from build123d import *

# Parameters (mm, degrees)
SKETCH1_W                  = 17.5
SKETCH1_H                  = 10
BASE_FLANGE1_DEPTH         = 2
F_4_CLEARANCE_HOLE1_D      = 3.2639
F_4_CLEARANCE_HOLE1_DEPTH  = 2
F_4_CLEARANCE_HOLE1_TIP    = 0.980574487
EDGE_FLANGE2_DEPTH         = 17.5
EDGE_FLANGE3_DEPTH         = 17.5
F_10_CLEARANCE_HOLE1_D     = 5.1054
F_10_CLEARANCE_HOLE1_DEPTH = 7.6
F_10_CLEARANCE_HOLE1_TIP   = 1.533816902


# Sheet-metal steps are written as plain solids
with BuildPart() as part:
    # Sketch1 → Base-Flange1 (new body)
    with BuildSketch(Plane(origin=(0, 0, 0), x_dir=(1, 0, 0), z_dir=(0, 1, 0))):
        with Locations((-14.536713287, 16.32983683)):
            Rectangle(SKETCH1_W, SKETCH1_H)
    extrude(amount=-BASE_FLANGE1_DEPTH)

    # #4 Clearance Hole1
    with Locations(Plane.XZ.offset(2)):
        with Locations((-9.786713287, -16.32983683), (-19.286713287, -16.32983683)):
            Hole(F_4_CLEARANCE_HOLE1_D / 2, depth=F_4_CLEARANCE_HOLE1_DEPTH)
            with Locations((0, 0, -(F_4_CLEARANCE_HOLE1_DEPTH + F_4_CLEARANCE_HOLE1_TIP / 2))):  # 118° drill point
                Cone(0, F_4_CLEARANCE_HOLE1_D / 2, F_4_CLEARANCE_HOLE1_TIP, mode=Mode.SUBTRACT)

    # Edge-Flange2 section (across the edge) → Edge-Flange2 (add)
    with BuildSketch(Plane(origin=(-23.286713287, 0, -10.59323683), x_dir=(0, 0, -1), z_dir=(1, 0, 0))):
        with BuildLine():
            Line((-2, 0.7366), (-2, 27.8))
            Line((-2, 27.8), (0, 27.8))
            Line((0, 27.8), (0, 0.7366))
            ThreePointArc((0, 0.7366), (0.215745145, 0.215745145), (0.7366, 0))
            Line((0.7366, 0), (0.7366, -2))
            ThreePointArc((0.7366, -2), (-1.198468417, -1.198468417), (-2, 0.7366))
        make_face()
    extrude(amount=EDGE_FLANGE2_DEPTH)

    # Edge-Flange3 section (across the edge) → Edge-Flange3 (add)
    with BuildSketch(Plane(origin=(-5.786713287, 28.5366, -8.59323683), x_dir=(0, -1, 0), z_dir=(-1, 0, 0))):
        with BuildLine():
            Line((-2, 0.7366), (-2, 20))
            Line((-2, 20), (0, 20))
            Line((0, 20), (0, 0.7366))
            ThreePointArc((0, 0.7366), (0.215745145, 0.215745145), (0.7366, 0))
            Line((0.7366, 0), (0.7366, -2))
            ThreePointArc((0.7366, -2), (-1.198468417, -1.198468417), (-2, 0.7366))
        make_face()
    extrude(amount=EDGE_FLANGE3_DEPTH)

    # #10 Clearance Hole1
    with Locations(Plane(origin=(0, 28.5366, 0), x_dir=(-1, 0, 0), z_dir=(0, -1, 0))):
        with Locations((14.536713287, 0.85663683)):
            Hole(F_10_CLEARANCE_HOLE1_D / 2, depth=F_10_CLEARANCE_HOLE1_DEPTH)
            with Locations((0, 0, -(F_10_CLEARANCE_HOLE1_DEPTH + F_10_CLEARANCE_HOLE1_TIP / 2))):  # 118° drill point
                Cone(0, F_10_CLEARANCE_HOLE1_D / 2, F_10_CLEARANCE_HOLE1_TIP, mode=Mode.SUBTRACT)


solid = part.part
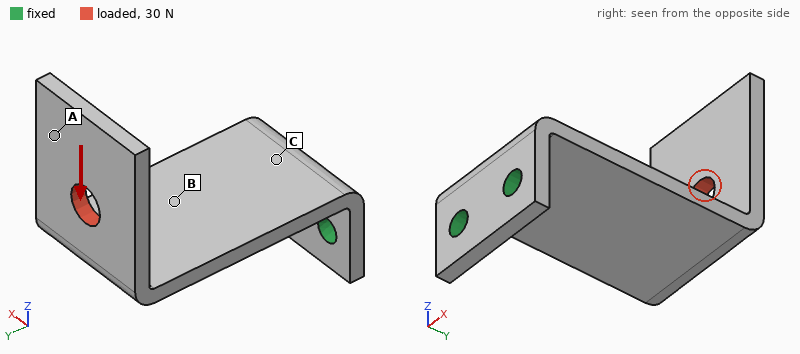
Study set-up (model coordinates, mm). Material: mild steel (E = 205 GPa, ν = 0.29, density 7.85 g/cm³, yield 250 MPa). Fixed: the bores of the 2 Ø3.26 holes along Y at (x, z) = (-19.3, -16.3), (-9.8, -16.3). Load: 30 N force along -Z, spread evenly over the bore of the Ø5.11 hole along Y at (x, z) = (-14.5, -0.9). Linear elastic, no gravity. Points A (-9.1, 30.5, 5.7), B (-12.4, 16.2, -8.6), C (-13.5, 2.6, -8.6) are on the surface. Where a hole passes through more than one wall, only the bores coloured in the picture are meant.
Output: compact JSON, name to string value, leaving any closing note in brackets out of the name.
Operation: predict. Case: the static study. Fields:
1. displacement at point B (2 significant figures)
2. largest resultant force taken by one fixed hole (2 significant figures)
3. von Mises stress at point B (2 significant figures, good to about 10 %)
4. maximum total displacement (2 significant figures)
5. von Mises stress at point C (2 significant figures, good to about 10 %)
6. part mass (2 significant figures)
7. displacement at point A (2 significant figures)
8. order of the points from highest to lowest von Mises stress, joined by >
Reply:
{"displacement at point B": "0.077 mm", "largest resultant force taken by one fixed hole": "20 N", "von Mises stress at point B": "33 MPa", "maximum total displacement": "0.24 mm", "von Mises stress at point C": "63 MPa", "part mass": "16 g", "displacement at point A": "0.22 mm", "order of the points from highest to lowest von Mises stress, joined by >": "C > B > A"}
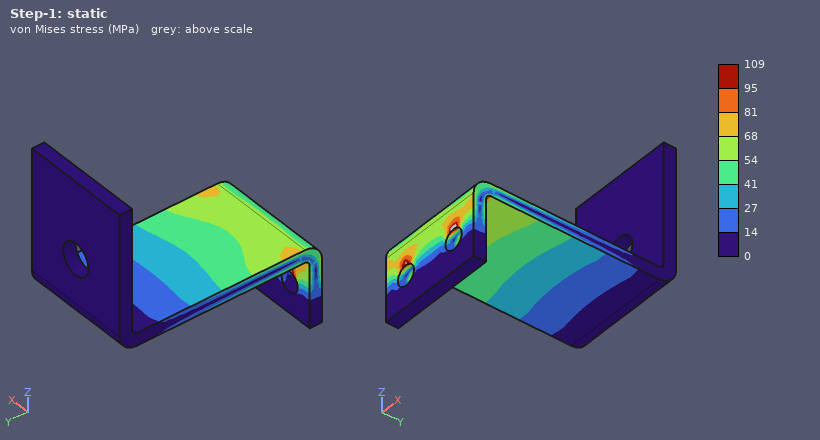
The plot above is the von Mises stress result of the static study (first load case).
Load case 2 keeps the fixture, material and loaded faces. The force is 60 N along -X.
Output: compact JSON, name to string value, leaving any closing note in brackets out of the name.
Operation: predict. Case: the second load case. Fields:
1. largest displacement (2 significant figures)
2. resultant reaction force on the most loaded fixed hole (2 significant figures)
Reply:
{"largest displacement": "96 µm", "resultant reaction force on the most loaded fixed hole": "180 N"}
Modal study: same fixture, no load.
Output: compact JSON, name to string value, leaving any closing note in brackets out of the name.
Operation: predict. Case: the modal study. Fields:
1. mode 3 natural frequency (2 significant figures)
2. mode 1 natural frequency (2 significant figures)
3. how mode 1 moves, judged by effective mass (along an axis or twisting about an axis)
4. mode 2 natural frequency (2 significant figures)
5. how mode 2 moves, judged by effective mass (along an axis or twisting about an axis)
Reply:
{"mode 3 natural frequency": "2500 Hz", "mode 1 natural frequency": "690 Hz", "how mode 1 moves, judged by effective mass": "along Z", "mode 2 natural frequency": "1800 Hz", "how mode 2 moves, judged by effective mass": "along X"}
